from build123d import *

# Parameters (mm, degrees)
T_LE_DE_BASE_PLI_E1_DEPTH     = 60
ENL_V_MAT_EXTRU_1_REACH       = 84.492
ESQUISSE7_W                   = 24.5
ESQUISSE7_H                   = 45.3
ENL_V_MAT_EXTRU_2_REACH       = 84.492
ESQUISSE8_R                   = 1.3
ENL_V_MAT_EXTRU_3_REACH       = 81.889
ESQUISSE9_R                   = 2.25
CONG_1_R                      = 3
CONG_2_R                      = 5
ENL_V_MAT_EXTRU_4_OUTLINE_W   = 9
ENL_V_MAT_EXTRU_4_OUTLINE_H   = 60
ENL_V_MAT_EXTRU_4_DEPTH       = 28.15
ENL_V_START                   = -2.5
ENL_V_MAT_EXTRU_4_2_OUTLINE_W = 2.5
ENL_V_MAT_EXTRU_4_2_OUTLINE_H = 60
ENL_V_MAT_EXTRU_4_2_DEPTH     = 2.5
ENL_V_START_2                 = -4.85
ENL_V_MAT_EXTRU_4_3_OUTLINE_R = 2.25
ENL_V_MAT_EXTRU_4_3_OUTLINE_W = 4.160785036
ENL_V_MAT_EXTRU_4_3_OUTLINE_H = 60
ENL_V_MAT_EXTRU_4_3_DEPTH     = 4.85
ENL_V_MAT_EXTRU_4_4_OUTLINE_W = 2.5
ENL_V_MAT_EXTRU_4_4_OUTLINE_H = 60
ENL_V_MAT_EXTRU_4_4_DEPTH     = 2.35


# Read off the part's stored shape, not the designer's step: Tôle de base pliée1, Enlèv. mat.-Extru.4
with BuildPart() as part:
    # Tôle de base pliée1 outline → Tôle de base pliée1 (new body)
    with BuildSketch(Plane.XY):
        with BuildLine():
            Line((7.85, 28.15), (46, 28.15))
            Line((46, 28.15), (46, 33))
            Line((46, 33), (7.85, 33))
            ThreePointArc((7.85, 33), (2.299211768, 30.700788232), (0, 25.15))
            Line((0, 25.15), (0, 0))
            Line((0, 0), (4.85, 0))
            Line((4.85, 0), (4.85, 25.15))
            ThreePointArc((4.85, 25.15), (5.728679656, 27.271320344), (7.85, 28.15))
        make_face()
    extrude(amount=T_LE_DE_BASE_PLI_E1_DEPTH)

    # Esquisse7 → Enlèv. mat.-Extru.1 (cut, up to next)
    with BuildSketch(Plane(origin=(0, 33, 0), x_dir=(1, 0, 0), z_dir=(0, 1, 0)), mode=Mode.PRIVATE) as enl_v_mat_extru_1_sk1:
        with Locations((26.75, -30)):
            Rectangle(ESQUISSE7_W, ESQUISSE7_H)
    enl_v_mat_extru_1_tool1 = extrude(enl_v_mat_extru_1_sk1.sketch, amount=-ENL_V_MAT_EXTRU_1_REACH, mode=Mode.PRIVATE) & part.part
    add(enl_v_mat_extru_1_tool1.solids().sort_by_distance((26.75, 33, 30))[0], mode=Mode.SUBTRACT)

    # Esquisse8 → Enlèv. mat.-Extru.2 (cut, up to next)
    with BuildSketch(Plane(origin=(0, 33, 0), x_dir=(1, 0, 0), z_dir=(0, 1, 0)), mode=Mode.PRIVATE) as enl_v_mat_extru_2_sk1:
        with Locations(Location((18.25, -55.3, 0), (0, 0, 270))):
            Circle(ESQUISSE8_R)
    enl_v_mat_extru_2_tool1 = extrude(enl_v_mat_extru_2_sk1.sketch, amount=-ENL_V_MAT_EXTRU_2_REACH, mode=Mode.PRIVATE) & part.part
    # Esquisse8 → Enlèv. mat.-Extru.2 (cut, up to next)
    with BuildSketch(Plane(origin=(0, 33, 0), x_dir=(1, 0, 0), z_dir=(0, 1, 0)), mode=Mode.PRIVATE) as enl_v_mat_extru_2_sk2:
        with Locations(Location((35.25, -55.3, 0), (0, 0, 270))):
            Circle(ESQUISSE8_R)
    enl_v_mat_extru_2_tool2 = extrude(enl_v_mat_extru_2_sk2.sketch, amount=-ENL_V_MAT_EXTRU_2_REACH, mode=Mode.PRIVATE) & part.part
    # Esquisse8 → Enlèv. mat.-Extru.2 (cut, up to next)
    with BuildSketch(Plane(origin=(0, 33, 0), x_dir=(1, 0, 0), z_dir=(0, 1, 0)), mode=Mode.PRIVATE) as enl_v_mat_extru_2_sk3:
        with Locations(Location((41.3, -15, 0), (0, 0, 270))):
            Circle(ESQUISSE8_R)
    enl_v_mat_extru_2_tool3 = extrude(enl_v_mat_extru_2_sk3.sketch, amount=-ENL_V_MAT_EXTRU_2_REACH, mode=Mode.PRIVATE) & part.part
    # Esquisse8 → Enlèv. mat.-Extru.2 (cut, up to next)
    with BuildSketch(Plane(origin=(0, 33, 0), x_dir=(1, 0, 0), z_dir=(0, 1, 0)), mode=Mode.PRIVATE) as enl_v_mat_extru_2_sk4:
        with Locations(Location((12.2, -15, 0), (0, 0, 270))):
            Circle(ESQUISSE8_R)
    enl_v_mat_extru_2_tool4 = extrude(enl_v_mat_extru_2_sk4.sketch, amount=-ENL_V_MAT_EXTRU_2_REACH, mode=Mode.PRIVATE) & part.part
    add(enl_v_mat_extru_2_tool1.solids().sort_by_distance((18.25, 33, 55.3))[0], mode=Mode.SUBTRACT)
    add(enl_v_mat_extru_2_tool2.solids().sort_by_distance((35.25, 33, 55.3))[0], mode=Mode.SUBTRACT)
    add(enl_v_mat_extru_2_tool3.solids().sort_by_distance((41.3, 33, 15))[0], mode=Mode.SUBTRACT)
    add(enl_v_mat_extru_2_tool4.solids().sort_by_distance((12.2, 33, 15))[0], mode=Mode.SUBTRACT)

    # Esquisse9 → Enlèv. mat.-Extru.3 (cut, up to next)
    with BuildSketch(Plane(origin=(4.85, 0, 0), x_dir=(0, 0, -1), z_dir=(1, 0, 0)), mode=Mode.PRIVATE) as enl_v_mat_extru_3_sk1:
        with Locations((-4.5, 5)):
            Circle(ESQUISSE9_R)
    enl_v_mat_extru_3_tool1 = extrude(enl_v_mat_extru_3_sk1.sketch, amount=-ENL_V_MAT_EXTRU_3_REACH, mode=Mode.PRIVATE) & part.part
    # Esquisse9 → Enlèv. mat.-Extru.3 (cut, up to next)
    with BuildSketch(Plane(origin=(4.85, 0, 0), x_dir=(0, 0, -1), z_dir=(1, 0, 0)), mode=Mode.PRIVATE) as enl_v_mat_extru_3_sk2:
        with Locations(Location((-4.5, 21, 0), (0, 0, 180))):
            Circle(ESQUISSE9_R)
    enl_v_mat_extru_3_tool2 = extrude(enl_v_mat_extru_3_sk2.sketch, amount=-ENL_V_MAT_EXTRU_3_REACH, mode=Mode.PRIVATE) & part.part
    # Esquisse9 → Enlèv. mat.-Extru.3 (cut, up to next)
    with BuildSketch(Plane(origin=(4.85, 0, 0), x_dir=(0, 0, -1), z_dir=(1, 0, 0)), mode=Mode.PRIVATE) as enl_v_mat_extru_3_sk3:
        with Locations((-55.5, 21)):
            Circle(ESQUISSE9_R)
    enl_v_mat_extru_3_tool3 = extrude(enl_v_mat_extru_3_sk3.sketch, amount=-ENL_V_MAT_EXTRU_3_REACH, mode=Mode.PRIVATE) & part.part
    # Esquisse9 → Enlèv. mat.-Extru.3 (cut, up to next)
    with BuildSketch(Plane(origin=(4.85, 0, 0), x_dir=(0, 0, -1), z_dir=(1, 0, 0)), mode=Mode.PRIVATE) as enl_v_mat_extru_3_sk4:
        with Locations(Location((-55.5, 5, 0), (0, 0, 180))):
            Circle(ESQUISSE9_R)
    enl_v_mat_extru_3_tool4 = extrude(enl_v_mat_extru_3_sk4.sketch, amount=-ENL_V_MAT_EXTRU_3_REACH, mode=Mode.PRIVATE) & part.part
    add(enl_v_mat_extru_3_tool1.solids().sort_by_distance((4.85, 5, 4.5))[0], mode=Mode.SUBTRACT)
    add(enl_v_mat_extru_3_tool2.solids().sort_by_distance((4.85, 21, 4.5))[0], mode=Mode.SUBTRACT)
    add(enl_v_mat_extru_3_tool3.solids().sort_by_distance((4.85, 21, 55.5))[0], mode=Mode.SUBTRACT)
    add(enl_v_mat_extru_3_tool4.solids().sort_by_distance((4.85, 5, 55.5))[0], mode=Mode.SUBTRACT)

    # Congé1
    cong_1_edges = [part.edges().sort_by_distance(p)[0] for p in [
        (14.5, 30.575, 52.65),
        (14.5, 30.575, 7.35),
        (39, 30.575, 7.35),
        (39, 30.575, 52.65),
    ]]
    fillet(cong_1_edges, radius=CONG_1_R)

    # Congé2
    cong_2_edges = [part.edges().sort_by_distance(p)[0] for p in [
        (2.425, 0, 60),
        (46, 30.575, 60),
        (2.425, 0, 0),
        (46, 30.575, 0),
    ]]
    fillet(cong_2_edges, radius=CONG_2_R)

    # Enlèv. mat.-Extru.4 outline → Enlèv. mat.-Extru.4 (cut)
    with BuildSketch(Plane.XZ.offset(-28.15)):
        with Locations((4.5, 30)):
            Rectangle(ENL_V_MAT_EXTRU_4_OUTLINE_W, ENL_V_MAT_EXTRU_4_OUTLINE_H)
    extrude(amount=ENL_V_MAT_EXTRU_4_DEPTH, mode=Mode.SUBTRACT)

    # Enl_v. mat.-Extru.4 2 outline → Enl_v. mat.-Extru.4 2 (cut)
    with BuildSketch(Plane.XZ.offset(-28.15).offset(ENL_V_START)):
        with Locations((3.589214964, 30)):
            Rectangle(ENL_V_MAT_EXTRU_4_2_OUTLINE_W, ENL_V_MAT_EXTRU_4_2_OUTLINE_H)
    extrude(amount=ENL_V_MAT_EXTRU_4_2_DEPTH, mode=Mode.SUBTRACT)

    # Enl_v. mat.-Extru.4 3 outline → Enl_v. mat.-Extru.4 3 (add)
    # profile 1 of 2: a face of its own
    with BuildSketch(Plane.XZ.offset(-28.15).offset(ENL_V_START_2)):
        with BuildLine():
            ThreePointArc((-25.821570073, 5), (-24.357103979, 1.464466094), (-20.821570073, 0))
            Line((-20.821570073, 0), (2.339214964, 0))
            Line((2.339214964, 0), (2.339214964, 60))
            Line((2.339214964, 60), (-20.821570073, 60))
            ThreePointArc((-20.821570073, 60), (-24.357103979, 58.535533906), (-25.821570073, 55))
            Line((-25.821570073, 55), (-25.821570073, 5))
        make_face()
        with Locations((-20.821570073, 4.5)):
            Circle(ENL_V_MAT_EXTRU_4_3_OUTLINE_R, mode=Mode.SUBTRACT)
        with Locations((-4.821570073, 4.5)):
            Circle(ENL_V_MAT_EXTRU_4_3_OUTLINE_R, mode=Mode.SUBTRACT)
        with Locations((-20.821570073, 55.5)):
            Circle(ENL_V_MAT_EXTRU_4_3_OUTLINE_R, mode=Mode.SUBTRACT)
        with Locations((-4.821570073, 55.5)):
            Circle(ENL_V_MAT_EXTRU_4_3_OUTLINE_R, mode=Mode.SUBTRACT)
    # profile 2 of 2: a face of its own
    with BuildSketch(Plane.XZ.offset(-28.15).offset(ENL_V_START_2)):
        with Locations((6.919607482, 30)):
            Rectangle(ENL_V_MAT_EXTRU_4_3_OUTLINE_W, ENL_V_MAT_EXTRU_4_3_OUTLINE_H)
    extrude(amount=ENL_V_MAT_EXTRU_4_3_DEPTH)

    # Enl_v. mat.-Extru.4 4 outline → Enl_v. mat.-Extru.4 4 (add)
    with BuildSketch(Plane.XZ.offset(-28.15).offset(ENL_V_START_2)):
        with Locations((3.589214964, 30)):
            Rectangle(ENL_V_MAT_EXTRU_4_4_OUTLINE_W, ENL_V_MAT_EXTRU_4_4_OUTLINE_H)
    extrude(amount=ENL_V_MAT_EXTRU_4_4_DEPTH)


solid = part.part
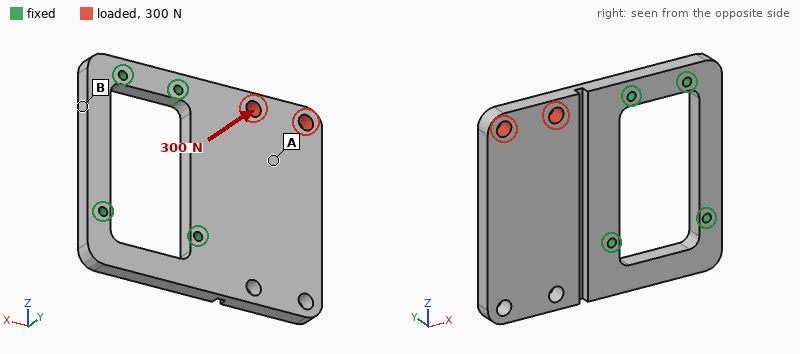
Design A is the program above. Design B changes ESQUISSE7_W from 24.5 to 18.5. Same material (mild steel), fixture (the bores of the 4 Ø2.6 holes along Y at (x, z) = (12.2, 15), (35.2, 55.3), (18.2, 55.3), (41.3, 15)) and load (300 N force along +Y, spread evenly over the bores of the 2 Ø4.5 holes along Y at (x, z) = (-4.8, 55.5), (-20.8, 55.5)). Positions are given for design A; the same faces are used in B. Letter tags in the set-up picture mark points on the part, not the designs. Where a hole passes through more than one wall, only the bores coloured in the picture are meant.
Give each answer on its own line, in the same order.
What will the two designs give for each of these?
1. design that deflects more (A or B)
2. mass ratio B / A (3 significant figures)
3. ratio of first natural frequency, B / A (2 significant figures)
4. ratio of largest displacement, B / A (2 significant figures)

A
1.09
1.0
0.92
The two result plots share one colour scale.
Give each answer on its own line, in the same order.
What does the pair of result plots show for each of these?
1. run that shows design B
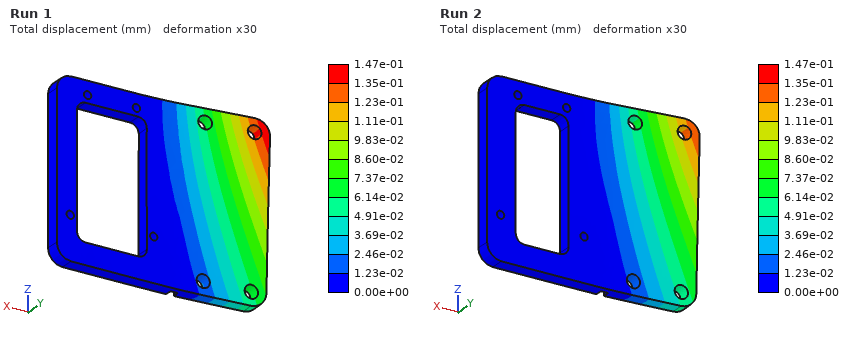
Run 2
